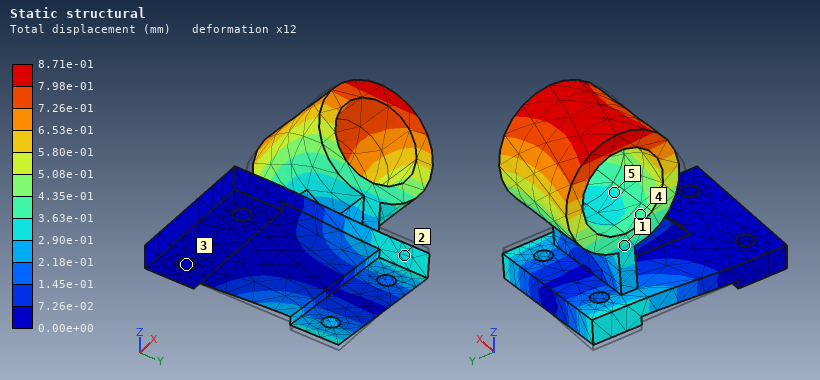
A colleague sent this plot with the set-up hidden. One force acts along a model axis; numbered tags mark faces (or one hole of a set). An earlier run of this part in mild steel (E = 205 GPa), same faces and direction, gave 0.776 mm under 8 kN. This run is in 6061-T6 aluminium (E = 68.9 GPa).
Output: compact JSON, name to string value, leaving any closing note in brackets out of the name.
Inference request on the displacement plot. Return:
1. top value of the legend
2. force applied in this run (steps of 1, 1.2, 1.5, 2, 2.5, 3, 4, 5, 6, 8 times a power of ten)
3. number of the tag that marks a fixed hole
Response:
{"top value of the legend": "8.71e-01 mm", "force applied in this run": "3 kN", "number of the tag that marks a fixed hole": "3"}
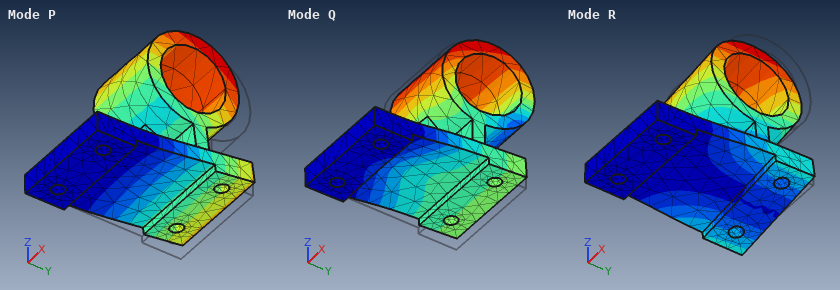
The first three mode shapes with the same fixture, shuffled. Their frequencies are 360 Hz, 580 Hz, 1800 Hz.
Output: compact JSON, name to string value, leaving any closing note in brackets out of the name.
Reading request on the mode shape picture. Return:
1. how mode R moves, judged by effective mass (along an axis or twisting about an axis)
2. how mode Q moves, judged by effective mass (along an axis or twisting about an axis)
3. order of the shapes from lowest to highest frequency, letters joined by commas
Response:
{"how mode R moves, judged by effective mass": "along X", "how mode Q moves, judged by effective mass": "along Z", "order of the shapes from lowest to highest frequency, letters joined by commas": "P, R, Q"}
